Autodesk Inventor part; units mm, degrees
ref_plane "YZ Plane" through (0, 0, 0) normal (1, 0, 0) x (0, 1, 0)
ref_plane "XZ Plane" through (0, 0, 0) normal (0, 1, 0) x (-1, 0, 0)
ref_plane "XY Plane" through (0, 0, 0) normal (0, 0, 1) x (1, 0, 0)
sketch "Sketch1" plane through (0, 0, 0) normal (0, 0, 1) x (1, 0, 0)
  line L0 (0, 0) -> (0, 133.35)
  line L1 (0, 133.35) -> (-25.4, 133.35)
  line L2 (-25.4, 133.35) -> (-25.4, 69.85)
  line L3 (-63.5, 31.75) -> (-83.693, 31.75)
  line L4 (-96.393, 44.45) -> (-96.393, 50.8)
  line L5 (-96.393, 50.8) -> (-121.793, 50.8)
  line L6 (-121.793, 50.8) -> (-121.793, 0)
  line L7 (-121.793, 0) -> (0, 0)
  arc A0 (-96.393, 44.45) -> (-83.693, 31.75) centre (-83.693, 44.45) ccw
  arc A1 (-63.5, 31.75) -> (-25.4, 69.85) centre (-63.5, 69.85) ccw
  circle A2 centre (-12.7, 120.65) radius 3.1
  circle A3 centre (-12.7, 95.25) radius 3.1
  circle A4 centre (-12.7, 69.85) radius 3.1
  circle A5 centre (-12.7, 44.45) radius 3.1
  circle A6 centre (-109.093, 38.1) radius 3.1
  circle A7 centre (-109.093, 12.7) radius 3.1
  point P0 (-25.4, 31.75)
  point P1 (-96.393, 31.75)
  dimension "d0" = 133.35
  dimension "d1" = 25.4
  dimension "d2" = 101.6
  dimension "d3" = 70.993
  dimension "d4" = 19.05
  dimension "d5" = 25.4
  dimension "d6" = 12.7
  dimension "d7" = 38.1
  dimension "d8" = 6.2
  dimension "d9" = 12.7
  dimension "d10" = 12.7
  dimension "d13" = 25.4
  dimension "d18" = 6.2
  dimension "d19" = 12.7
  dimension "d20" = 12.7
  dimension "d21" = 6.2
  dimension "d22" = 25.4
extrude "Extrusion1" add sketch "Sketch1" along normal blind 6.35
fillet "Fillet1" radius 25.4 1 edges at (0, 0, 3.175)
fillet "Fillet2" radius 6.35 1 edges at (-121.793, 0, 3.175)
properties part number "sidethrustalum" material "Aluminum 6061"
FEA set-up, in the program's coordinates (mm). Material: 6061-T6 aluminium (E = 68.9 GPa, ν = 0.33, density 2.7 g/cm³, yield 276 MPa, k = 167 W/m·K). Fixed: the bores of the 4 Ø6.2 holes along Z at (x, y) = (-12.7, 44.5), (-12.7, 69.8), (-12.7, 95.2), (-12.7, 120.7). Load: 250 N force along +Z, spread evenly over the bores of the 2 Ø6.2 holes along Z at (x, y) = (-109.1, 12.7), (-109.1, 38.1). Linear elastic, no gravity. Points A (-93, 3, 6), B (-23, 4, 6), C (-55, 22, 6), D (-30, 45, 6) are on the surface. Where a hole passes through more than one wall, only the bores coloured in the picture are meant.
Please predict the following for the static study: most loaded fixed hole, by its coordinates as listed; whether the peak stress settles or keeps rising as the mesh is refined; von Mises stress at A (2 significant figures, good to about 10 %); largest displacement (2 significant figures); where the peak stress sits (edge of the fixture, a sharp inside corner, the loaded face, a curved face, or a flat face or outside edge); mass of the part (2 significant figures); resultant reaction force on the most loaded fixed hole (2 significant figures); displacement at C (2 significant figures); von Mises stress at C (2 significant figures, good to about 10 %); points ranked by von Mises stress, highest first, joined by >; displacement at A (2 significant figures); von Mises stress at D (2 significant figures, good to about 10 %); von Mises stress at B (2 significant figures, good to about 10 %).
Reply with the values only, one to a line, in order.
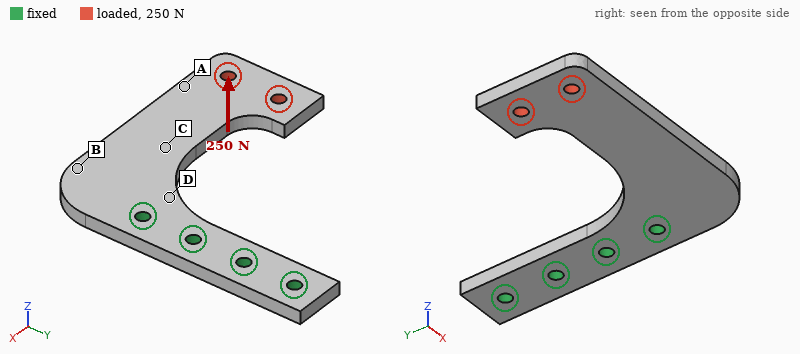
(-12.7, 44.5)
keeps rising
19 MPa
1.9 mm
edge of the fixture
120 g
380 N
0.44 mm
66 MPa
D > C > B > A
1.2 mm
88 MPa
41 MPa
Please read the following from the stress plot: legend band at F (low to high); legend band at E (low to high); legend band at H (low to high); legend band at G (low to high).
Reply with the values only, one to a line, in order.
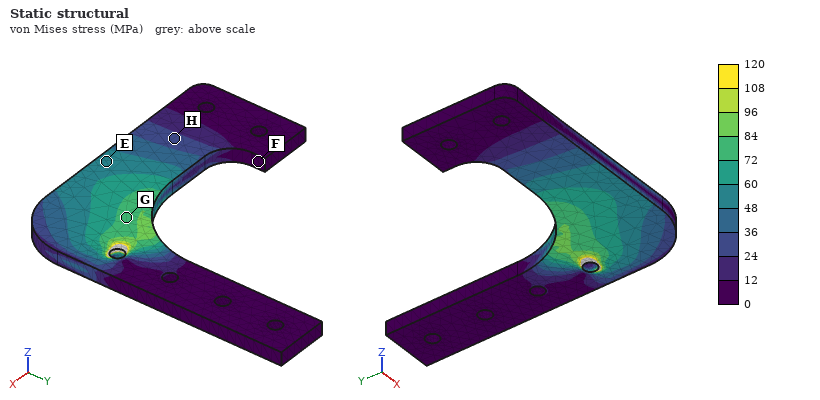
0 to 12 MPa
48 to 60 MPa
24 to 36 MPa
72 to 84 MPa
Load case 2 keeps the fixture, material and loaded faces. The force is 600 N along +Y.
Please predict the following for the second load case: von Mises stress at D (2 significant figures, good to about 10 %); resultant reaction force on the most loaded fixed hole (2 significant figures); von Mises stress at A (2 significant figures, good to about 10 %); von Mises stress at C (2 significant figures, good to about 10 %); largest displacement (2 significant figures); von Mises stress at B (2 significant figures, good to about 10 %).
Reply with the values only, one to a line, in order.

35 MPa
1.6 kN
7.5 MPa
10 MPa
0.25 mm
13 MPa
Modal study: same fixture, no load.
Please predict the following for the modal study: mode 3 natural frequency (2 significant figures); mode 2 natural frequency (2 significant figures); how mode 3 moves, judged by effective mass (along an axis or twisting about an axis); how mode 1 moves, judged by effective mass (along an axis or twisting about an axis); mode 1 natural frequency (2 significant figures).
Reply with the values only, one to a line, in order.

1500 Hz
1300 Hz
along Y
along Z
370 Hz
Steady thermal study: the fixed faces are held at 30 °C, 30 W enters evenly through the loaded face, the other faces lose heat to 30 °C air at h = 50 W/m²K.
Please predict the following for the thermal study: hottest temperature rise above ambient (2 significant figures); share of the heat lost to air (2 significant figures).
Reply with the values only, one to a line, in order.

55 K
53 %
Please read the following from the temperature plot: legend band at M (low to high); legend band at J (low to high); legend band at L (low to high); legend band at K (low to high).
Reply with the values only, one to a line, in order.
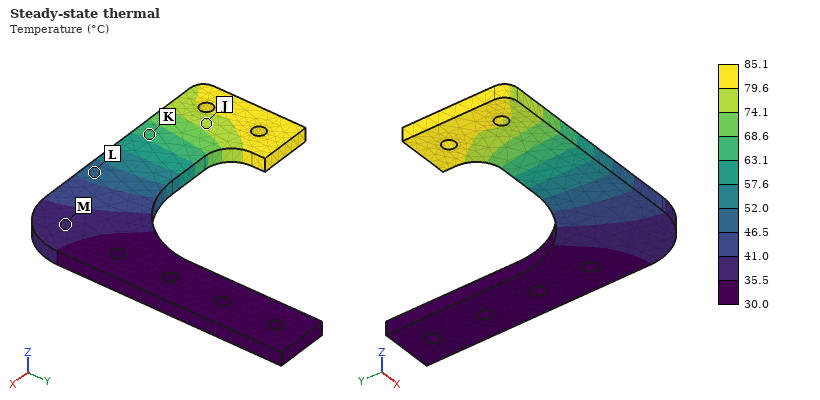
35.5 to 41.0 °C
74.1 to 79.6 °C
46.5 to 52.0 °C
63.1 to 68.6 °C
